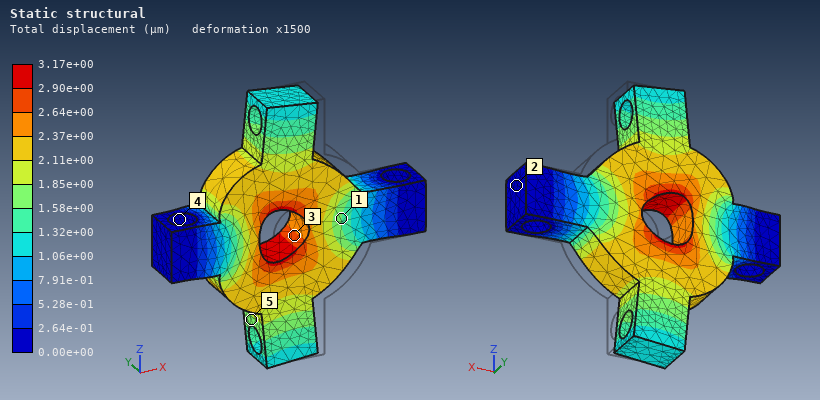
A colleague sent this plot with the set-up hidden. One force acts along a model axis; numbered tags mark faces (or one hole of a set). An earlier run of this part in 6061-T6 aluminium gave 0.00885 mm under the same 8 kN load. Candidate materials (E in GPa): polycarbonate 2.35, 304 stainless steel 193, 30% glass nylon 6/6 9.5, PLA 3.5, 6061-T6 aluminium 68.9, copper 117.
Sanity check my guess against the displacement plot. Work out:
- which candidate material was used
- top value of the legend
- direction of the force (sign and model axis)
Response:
304 stainless steel
3.17e+00 µm
-X
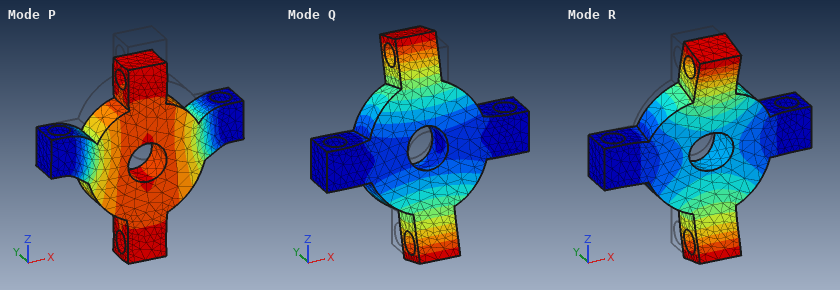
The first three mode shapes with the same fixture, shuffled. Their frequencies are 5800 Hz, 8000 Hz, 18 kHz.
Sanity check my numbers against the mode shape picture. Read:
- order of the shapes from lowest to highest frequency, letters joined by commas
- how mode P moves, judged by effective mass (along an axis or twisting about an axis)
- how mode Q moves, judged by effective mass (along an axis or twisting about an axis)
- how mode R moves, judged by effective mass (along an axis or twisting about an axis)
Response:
Q, R, P
along Z
twisting about X
along Y
